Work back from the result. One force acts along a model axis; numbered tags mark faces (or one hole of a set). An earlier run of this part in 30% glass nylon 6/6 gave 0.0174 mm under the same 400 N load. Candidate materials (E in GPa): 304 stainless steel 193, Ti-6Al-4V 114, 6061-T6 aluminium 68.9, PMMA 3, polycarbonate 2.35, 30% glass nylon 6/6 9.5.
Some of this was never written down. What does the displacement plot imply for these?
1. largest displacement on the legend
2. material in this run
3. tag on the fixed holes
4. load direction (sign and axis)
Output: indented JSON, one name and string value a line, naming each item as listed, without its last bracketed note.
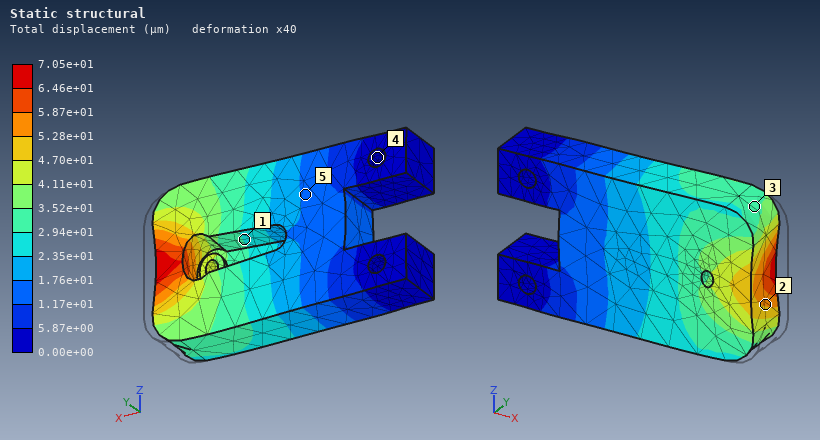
{
  "largest displacement on the legend": "7.05e+01 µm",
  "material in this run": "polycarbonate",
  "tag on the fixed holes": "4",
  "load direction": "-X"
}
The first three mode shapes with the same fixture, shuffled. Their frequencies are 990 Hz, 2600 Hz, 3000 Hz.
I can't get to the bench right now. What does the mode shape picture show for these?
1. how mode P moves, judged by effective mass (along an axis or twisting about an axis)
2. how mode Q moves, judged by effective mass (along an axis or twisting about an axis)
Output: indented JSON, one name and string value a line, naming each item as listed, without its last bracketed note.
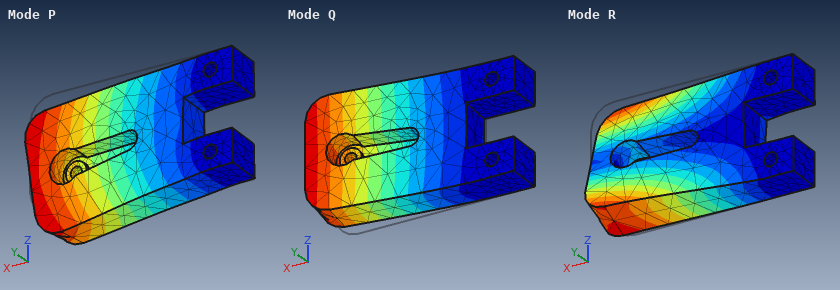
{
  "how mode P moves, judged by effective mass": "along Z",
  "how mode Q moves, judged by effective mass": "along Y"
}
